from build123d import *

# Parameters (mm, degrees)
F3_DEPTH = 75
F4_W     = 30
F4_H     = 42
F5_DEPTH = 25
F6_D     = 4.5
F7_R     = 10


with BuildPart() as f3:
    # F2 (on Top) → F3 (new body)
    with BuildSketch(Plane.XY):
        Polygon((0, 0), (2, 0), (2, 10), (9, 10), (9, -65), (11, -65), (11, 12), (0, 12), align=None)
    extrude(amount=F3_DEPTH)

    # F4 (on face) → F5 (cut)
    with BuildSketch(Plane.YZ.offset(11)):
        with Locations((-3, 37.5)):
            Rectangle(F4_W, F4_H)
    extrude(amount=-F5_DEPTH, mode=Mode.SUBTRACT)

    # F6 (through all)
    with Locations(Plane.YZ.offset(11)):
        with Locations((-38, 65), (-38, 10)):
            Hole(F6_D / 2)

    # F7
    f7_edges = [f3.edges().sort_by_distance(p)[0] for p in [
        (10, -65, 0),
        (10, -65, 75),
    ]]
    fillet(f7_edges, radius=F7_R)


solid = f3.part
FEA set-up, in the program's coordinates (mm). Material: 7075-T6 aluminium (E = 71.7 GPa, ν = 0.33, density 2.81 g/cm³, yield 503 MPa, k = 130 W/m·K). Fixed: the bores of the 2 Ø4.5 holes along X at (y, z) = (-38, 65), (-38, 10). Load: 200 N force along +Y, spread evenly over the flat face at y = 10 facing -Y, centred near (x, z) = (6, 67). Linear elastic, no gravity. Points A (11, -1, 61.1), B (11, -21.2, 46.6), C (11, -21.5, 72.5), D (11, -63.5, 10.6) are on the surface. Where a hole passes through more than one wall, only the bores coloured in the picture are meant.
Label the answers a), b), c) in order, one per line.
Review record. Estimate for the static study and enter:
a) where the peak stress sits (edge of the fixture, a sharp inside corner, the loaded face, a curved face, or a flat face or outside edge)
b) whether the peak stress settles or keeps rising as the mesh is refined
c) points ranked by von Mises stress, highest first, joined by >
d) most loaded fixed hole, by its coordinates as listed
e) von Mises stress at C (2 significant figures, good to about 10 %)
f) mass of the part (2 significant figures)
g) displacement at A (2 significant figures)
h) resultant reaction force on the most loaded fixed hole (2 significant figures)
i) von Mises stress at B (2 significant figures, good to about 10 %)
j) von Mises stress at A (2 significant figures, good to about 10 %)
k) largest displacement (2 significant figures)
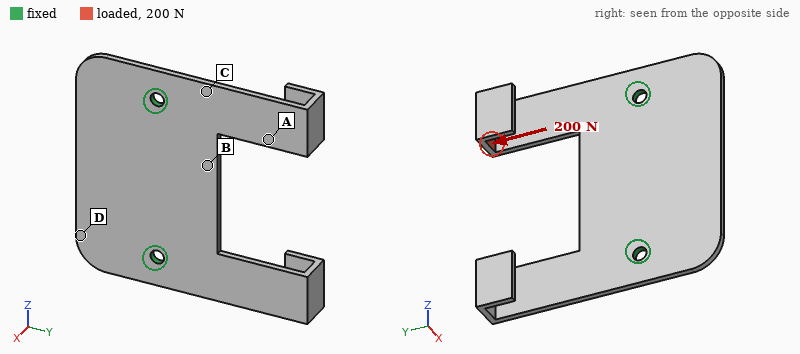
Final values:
a) a sharp inside corner
b) keeps rising
c) A > C > B > D
d) (-38, 65)
e) 60 MPa
f) 28 g
g) 0.52 mm
h) 200 N
i) 24 MPa
j) 76 MPa
k) 1.2 mm
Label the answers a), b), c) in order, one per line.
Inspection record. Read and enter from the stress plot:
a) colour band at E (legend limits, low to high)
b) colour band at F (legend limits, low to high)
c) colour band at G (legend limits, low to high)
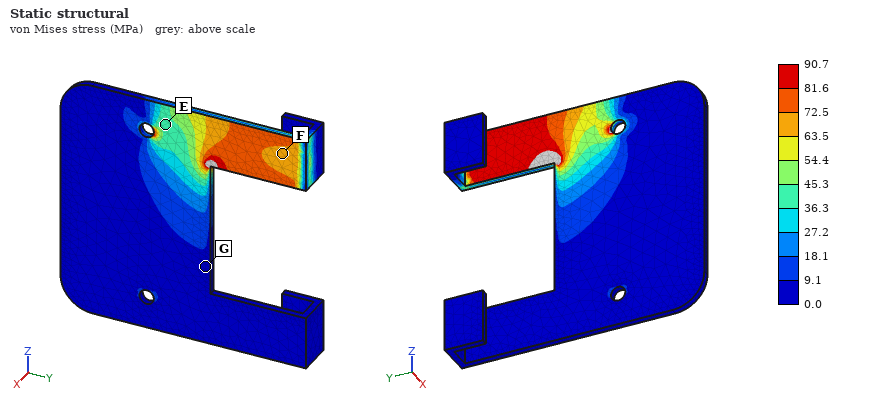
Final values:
a) 36.3 to 45.3 MPa
b) 63.5 to 72.5 MPa
c) 0.0 to 9.1 MPa
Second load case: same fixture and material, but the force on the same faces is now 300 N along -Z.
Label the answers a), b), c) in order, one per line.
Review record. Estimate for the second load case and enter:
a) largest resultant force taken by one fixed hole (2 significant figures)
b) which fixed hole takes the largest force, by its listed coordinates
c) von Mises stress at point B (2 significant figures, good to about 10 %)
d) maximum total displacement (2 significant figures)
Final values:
a) 310 N
b) (-38, 10)
c) 16 MPa
d) 0.78 mm
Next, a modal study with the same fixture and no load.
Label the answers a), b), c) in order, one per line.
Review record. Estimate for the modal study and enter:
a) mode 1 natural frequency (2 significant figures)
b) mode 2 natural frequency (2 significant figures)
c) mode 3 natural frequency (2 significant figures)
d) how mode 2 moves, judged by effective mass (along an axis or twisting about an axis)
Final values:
a) 520 Hz
b) 540 Hz
c) 1800 Hz
d) twisting about Y
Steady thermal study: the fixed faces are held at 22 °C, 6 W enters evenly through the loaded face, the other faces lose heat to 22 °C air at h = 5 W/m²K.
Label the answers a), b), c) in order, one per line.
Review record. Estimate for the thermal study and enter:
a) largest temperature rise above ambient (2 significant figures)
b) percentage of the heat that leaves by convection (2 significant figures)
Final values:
a) 62 K
b) 8.7 %
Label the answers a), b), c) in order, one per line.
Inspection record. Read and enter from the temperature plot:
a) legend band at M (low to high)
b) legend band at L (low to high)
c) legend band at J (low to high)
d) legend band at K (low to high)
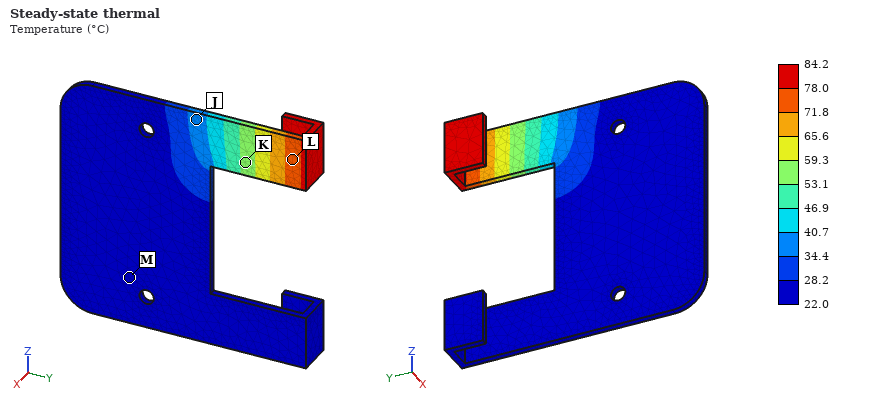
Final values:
a) 22.0 to 28.2 °C
b) 71.8 to 78.0 °C
c) 34.4 to 40.7 °C
d) 53.1 to 59.3 °C
